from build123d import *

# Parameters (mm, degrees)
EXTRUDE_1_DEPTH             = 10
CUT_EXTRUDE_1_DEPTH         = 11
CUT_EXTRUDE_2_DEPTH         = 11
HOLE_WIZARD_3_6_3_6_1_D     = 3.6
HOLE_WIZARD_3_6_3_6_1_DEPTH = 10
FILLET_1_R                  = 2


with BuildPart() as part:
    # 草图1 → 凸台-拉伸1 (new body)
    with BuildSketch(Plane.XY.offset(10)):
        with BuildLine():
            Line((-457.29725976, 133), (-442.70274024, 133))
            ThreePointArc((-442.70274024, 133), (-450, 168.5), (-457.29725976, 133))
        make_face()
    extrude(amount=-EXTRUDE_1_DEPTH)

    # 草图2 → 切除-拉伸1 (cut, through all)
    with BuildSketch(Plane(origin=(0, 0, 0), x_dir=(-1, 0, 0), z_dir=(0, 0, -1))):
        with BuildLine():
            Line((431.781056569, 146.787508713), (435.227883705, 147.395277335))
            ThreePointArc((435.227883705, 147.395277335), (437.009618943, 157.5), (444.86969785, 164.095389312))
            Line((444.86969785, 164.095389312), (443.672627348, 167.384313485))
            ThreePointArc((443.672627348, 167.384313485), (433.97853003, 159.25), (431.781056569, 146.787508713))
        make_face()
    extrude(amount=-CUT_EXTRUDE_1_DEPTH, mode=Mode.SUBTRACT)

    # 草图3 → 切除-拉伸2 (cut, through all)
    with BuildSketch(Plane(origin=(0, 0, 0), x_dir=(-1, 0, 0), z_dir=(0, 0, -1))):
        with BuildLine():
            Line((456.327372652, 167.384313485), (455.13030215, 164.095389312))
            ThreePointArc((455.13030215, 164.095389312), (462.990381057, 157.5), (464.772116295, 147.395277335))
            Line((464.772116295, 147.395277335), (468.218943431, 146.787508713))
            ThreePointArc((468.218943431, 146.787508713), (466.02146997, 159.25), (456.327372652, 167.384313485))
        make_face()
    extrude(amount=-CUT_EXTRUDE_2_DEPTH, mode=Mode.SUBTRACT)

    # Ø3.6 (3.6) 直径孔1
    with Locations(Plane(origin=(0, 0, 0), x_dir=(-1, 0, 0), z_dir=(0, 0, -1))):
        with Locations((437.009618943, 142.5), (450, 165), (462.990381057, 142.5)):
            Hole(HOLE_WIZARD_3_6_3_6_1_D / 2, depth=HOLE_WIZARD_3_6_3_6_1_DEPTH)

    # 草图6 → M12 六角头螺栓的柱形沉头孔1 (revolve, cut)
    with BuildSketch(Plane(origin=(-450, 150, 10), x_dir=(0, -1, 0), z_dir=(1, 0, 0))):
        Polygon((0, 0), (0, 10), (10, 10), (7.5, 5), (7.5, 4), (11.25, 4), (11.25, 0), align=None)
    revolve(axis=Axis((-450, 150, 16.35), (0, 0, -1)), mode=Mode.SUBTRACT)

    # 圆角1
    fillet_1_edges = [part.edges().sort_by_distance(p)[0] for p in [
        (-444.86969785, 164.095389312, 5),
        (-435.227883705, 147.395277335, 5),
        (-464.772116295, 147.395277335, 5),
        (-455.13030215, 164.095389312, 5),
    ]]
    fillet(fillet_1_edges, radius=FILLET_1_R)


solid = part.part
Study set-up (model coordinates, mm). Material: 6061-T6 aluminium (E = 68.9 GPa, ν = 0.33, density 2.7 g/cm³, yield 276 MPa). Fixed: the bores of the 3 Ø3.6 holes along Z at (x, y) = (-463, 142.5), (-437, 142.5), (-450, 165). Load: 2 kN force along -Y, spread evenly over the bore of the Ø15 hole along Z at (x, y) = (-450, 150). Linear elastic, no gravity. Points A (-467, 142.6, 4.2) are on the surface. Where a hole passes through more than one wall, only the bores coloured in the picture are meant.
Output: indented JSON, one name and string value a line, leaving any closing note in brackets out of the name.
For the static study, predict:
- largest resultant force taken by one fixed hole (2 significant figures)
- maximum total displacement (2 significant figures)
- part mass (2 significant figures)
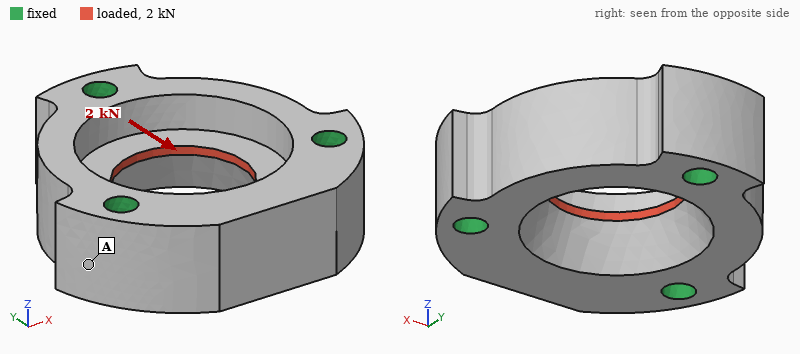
{
  "largest resultant force taken by one fixed hole": "740 N",
  "maximum total displacement": "4.7 µm",
  "part mass": "15 g"
}
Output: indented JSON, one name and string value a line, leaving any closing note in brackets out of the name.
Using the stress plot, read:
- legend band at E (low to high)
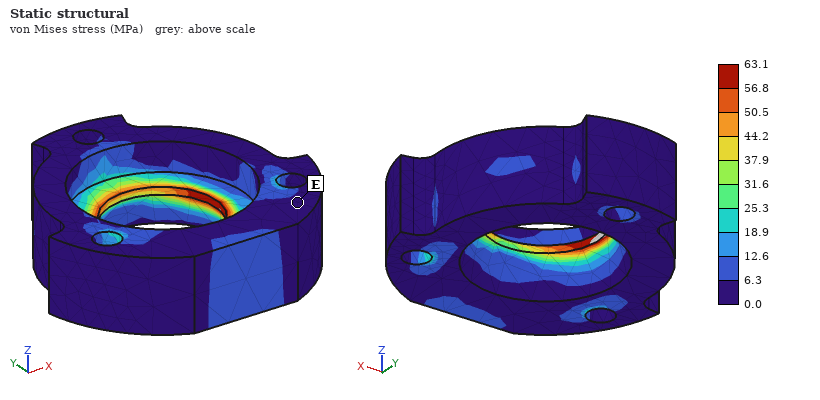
{
  "legend band at E": "0.0 to 6.3 MPa"
}
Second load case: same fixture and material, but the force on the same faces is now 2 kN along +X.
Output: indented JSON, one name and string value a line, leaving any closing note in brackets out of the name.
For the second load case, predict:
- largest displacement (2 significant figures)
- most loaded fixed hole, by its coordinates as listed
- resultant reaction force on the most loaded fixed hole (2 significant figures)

{
  "largest displacement": "5.1 µm",
  "most loaded fixed hole, by its coordinates as listed": "(-450, 165)",
  "resultant reaction force on the most loaded fixed hole": "800 N"
}
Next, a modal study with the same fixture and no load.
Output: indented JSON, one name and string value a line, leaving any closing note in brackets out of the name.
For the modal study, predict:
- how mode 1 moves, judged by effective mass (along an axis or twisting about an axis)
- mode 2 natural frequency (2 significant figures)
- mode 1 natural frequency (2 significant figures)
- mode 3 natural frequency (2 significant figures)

{
  "how mode 1 moves, judged by effective mass": "along Z",
  "mode 2 natural frequency": "43 kHz",
  "mode 1 natural frequency": "38 kHz",
  "mode 3 natural frequency": "44 kHz"
}
